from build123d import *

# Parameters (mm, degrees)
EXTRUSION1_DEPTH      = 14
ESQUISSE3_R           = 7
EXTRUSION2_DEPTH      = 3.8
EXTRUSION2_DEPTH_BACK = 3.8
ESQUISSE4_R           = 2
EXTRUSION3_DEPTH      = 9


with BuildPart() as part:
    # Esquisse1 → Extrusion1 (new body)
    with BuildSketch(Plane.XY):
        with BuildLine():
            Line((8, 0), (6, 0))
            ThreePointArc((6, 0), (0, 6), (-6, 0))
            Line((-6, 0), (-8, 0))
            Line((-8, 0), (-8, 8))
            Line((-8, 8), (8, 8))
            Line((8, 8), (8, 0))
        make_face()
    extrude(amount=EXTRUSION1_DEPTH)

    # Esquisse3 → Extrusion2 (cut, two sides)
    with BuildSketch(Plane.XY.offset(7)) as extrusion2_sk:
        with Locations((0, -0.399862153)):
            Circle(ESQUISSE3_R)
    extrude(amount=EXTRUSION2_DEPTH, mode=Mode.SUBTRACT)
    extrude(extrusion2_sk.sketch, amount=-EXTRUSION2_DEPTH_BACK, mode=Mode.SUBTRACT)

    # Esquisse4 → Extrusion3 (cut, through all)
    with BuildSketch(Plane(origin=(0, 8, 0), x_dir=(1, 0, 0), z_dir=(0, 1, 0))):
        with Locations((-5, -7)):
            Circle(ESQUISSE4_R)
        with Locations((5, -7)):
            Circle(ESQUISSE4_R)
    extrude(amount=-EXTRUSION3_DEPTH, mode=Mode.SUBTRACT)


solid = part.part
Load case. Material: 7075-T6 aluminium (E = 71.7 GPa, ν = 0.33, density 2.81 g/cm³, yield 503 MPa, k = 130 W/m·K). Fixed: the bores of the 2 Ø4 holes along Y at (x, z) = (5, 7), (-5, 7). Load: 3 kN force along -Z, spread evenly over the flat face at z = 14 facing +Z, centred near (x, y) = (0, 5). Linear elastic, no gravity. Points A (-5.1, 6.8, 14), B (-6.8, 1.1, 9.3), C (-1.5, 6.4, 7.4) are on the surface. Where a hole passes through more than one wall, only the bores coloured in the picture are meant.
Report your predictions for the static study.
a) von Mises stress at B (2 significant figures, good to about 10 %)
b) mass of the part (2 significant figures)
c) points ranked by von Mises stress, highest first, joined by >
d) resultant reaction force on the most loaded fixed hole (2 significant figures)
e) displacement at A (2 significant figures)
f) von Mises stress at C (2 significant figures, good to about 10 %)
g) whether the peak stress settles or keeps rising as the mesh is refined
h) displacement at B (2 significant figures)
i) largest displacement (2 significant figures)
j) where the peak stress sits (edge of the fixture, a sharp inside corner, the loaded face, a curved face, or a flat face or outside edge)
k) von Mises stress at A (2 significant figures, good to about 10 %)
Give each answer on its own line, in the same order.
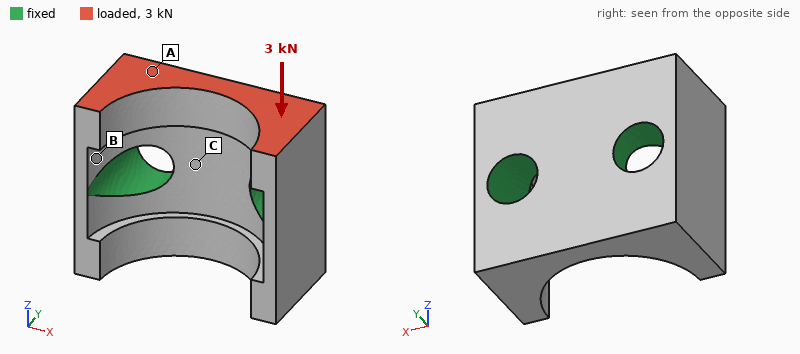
90 MPa
2.2 g
B > A > C
1.5 kN
3.9 µm
21 MPa
keeps rising
2.7 µm
8.8 µm
edge of the fixture
44 MPa
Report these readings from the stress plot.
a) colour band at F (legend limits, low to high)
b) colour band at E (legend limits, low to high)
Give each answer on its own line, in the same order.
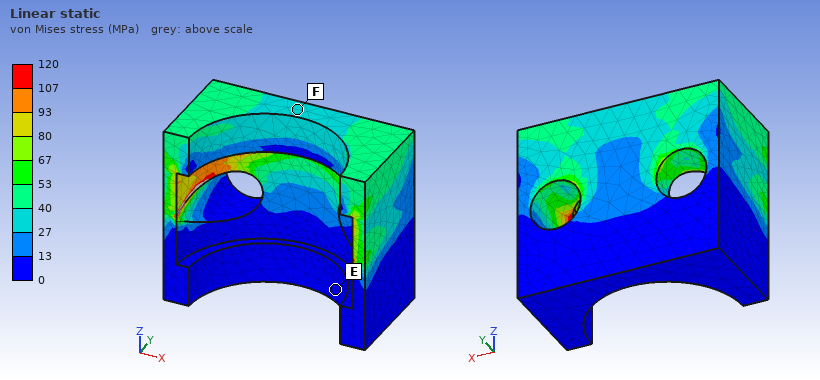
27 to 40 MPa
0 to 13 MPa
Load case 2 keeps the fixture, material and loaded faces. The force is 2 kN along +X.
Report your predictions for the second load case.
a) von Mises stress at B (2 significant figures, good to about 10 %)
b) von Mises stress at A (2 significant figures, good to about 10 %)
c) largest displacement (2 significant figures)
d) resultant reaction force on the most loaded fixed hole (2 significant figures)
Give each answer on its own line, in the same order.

86 MPa
88 MPa
41 µm
1.2 kN
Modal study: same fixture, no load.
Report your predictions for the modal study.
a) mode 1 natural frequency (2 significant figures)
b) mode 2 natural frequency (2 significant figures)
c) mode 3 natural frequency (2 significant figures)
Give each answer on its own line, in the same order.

65 kHz
66 kHz
67 kHz
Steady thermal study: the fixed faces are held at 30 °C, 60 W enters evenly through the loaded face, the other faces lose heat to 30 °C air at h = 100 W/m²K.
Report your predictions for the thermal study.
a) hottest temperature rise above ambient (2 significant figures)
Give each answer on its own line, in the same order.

44 K
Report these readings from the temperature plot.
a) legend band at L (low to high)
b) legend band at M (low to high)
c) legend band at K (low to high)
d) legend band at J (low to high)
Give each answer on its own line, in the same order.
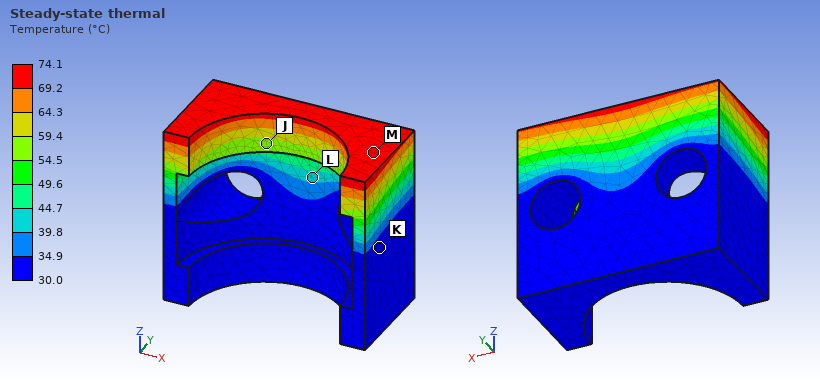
39.8 to 44.7 °C
69.2 to 74.1 °C
30.0 to 34.9 °C
54.5 to 59.4 °C
